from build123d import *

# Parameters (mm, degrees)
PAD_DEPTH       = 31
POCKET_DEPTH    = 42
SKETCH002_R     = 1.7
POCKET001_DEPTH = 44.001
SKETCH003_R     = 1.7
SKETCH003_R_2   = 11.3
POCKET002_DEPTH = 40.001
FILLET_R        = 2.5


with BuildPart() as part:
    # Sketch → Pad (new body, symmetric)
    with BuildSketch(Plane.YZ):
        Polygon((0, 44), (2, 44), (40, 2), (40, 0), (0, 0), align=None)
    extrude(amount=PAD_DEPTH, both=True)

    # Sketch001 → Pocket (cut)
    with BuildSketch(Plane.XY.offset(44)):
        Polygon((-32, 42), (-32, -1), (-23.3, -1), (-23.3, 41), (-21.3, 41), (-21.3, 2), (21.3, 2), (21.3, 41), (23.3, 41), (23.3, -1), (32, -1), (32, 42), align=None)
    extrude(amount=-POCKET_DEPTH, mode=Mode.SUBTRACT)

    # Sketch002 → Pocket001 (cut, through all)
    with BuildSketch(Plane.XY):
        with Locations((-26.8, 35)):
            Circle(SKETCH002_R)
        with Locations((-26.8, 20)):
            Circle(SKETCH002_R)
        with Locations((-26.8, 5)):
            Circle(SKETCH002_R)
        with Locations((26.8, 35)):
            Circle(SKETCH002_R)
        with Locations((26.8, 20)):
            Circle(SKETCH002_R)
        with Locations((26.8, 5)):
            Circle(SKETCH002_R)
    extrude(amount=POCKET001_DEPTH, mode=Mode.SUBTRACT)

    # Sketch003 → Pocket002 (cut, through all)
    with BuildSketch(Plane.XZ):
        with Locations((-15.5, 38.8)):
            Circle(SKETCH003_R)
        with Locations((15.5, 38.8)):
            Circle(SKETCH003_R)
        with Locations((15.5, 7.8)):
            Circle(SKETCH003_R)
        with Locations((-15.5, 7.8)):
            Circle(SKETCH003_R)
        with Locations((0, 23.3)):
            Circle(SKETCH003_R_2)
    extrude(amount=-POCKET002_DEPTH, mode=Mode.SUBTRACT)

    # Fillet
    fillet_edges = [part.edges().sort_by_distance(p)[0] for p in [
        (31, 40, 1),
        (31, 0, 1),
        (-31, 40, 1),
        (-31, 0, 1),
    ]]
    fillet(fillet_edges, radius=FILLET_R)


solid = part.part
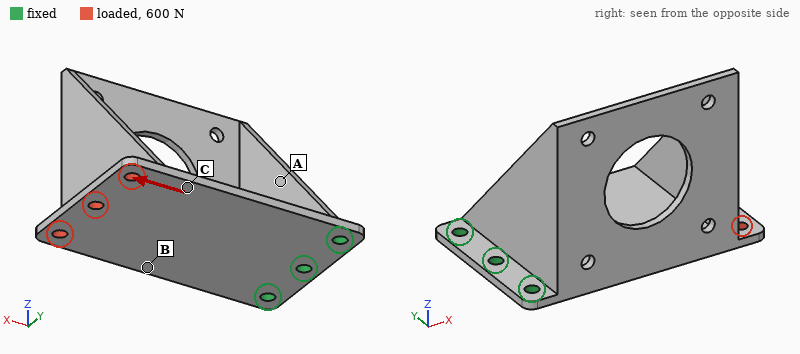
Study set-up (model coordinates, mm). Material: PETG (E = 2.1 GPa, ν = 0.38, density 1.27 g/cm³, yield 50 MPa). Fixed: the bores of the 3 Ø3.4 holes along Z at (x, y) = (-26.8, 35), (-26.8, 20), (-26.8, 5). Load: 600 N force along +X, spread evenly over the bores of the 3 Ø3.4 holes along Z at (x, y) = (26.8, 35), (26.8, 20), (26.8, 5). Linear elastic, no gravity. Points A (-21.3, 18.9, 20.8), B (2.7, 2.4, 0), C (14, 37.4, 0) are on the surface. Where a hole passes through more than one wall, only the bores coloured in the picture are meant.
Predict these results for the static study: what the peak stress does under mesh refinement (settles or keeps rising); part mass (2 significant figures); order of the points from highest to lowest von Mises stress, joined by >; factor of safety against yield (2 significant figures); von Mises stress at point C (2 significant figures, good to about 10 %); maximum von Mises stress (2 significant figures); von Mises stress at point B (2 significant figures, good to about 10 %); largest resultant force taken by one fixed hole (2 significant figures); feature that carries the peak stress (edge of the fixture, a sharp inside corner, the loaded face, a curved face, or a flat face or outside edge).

settles
14 g
C > B > A
1.9
8.6 MPa
26 MPa
5.2 MPa
210 N
the loaded face
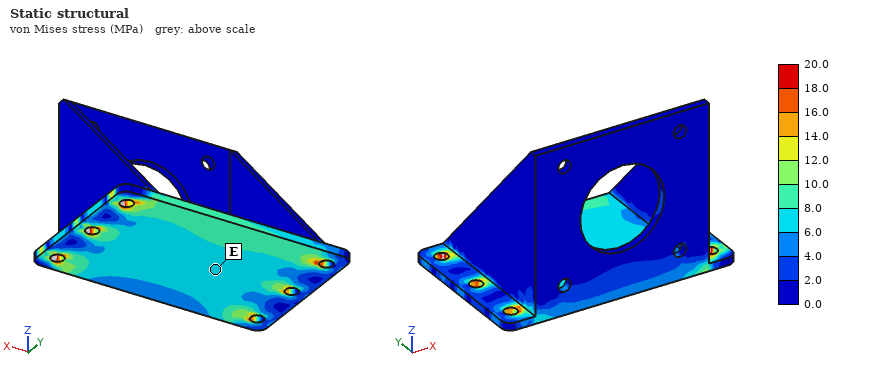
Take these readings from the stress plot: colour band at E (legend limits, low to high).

6.0 to 8.0 MPa
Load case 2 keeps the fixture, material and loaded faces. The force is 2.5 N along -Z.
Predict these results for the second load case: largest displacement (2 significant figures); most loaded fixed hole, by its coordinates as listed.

0.98 mm
(-26.8, 20)
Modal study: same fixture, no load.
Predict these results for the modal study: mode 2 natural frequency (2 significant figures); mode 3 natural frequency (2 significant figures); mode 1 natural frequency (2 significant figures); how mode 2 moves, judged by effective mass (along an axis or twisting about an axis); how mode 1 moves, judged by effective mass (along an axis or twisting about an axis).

250 Hz
860 Hz
110 Hz
along Y
along Z
